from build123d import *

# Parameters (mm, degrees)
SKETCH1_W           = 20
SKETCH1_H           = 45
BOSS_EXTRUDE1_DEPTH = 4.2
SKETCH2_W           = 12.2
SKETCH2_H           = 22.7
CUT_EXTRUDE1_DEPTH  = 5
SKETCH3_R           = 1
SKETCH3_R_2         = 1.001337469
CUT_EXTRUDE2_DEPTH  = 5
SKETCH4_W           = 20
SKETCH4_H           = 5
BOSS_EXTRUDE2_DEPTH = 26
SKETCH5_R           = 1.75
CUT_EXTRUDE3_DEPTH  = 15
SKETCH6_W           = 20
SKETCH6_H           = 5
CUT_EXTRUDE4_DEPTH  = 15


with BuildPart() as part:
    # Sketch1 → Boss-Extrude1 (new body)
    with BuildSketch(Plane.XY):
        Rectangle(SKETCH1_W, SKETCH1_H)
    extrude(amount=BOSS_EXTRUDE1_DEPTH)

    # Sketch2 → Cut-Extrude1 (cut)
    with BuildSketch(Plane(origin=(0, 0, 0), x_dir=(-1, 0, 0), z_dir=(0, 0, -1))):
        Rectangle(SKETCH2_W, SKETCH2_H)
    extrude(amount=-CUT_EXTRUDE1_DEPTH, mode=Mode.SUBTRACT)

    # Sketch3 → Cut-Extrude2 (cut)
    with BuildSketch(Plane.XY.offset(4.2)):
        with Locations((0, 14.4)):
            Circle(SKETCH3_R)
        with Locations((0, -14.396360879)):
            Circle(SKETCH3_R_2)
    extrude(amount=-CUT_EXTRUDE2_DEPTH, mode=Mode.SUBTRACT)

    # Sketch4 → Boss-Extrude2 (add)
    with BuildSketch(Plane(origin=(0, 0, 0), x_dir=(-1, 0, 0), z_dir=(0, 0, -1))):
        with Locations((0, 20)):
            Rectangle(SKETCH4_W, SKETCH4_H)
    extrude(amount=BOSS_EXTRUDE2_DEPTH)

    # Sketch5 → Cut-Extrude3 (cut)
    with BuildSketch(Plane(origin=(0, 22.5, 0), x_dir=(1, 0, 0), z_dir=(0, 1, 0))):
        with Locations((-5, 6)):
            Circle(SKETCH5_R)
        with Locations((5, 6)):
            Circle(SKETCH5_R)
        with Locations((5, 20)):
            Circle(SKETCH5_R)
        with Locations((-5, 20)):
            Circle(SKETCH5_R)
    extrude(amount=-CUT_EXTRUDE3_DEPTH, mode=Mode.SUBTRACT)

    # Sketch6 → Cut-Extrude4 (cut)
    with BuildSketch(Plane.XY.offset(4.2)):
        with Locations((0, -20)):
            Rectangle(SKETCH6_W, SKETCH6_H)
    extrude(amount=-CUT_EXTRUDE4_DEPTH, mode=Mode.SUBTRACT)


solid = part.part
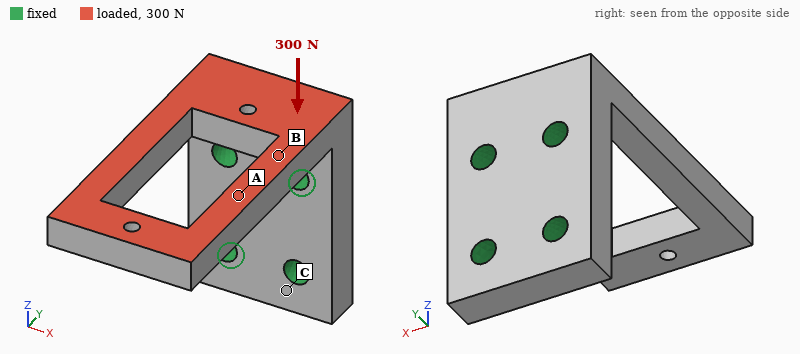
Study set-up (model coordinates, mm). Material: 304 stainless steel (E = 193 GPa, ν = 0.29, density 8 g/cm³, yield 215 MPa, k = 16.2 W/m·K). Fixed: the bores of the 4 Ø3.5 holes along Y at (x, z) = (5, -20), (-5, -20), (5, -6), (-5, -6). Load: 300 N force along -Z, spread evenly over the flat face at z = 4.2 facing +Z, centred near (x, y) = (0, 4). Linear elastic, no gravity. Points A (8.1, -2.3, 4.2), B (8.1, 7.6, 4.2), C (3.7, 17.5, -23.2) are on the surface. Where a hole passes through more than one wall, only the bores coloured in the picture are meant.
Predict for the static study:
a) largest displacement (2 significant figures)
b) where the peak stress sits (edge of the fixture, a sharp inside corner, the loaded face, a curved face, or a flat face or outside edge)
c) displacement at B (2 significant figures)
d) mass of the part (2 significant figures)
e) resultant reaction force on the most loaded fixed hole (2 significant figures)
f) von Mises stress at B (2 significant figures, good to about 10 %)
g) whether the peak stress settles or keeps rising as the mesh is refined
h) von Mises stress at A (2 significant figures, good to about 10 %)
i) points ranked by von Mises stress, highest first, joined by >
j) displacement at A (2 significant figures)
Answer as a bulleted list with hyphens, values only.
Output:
- 0.16 mm
- a sharp inside corner
- 0.028 mm
- 37 g
- 150 N
- 100 MPa
- keeps rising
- 45 MPa
- B > A > C
- 0.073 mm
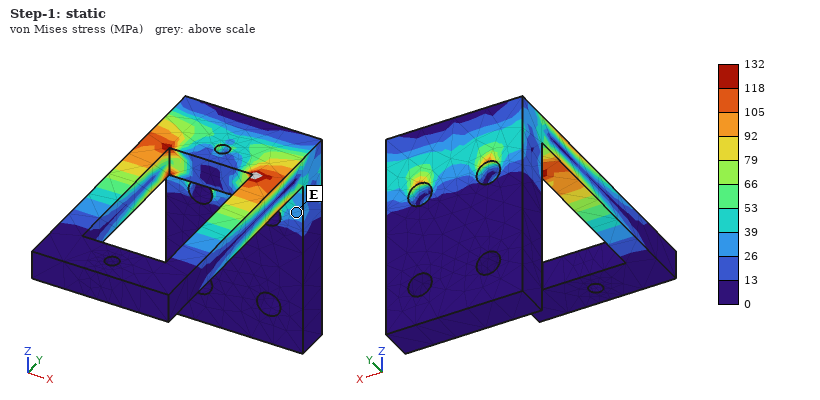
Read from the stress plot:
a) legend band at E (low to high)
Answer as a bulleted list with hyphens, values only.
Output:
- 26 to 39 MPa
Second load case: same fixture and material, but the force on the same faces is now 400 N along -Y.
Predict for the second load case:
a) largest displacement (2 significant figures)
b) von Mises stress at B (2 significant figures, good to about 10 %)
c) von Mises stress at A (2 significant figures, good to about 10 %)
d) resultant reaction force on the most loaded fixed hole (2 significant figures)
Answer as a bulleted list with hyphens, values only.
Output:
- 42 µm
- 25 MPa
- 18 MPa
- 220 N
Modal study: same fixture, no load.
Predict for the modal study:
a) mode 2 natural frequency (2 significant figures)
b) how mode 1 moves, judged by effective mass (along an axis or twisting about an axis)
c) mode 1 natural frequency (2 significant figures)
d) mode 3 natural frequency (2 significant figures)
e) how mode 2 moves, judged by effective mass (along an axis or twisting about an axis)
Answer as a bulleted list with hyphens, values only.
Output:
- 3600 Hz
- along Z
- 1900 Hz
- 5700 Hz
- along X
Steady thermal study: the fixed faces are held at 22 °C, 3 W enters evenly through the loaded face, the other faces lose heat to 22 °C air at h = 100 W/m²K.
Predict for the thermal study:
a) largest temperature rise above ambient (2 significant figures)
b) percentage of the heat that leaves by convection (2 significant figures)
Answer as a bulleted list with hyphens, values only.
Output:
- 19 K
- 58 %
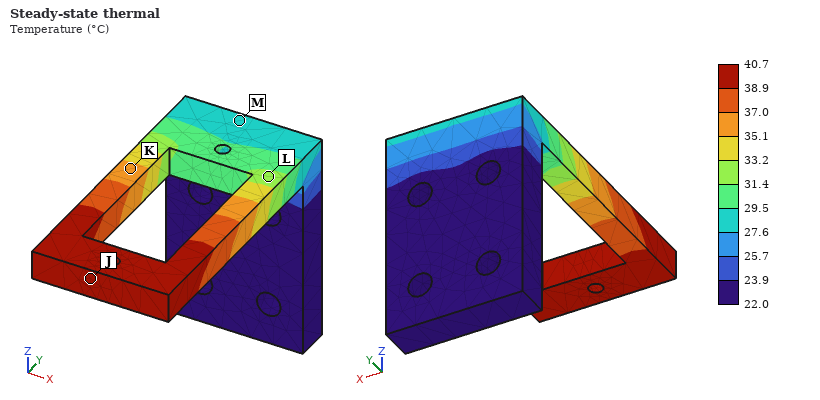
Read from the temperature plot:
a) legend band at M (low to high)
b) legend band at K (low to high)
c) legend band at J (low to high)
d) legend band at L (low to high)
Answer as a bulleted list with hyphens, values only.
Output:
- 27.6 to 29.5 °C
- 35.1 to 37.0 °C
- 38.9 to 40.7 °C
- 31.4 to 33.2 °C
